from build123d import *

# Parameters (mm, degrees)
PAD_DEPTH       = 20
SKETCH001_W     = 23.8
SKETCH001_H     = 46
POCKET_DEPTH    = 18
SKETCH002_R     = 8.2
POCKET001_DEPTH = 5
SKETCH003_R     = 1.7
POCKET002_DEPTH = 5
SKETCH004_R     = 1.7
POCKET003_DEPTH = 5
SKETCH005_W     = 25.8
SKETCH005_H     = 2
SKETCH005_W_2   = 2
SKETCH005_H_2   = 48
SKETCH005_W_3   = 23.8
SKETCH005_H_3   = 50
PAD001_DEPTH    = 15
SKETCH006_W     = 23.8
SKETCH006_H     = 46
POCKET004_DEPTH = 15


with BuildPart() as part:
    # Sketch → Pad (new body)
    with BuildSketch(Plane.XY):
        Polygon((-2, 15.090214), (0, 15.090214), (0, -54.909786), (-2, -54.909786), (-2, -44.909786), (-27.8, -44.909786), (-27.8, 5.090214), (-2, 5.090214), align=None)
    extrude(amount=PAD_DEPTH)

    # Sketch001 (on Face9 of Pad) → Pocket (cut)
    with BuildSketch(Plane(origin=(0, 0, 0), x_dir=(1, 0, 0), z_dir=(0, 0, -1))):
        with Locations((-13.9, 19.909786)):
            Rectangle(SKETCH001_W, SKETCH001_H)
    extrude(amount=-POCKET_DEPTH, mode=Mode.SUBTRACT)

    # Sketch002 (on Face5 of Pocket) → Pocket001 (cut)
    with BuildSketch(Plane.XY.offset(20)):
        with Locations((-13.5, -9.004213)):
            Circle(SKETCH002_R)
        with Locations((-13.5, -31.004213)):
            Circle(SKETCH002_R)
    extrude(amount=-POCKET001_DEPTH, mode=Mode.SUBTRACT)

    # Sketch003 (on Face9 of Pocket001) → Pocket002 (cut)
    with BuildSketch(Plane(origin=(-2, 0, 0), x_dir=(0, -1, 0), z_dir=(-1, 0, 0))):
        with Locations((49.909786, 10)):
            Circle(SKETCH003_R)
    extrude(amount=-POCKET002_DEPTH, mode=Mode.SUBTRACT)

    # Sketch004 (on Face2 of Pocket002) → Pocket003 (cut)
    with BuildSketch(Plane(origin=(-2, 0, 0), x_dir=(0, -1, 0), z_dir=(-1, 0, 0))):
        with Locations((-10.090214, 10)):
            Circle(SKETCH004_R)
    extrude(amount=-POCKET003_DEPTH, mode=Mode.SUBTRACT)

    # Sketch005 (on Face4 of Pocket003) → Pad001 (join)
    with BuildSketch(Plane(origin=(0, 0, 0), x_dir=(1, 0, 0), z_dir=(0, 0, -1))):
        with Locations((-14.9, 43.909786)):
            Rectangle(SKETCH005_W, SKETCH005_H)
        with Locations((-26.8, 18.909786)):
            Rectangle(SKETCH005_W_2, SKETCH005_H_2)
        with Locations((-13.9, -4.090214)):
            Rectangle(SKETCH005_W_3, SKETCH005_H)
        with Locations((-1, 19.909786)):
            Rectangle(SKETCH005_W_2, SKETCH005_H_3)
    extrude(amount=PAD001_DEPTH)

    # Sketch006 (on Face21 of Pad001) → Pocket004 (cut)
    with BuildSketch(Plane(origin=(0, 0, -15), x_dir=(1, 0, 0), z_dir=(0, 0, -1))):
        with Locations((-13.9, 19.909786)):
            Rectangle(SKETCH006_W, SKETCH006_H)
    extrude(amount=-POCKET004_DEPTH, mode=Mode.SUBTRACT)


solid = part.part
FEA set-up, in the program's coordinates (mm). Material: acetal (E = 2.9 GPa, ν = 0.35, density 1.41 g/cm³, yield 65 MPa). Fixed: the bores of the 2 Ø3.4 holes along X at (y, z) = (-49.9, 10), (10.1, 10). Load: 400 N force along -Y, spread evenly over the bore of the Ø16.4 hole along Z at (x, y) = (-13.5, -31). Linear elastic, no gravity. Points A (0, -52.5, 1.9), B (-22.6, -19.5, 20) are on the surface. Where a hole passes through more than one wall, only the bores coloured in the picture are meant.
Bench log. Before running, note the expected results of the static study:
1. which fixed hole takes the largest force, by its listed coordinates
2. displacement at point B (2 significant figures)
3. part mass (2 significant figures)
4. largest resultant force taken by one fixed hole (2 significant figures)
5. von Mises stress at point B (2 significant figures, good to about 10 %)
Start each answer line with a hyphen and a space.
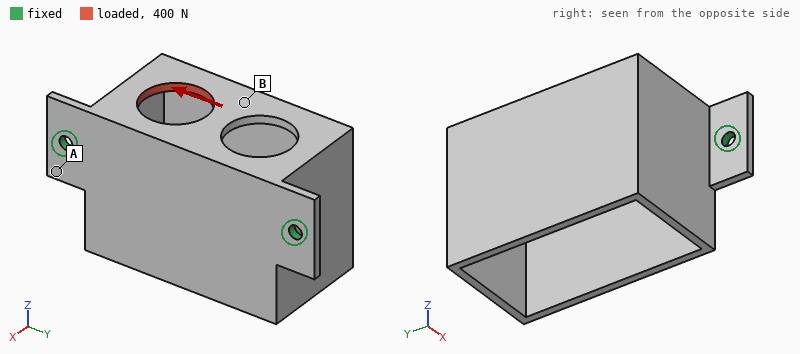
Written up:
- (-49.9, 10)
- 0.36 mm
- 18 g
- 250 N
- 7.5 MPa
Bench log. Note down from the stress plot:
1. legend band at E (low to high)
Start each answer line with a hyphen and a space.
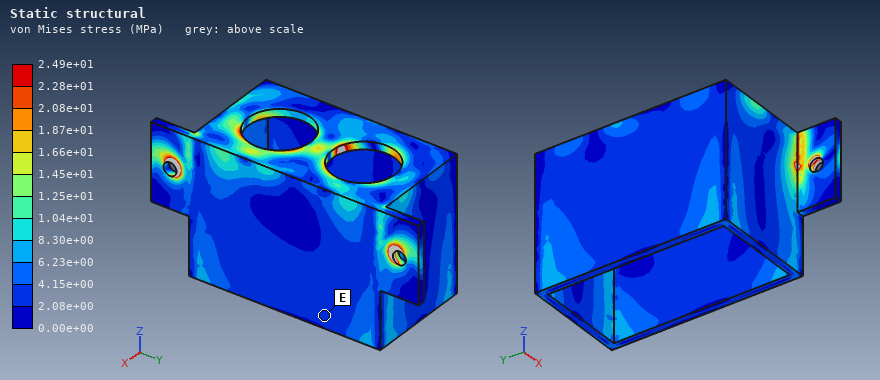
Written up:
- 2.08e+00 to 4.15e+00 MPa
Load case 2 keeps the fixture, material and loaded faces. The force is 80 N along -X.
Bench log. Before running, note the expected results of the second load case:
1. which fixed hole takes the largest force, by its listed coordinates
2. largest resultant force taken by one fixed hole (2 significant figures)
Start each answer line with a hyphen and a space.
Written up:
- (-49.9, 10)
- 59 N
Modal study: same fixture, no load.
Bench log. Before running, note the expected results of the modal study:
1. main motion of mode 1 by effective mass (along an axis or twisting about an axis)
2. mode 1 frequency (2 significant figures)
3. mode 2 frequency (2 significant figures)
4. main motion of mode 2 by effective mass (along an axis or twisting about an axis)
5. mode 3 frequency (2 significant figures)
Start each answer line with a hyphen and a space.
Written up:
- along Z
- 310 Hz
- 580 Hz
- along Y
- 1100 Hz
